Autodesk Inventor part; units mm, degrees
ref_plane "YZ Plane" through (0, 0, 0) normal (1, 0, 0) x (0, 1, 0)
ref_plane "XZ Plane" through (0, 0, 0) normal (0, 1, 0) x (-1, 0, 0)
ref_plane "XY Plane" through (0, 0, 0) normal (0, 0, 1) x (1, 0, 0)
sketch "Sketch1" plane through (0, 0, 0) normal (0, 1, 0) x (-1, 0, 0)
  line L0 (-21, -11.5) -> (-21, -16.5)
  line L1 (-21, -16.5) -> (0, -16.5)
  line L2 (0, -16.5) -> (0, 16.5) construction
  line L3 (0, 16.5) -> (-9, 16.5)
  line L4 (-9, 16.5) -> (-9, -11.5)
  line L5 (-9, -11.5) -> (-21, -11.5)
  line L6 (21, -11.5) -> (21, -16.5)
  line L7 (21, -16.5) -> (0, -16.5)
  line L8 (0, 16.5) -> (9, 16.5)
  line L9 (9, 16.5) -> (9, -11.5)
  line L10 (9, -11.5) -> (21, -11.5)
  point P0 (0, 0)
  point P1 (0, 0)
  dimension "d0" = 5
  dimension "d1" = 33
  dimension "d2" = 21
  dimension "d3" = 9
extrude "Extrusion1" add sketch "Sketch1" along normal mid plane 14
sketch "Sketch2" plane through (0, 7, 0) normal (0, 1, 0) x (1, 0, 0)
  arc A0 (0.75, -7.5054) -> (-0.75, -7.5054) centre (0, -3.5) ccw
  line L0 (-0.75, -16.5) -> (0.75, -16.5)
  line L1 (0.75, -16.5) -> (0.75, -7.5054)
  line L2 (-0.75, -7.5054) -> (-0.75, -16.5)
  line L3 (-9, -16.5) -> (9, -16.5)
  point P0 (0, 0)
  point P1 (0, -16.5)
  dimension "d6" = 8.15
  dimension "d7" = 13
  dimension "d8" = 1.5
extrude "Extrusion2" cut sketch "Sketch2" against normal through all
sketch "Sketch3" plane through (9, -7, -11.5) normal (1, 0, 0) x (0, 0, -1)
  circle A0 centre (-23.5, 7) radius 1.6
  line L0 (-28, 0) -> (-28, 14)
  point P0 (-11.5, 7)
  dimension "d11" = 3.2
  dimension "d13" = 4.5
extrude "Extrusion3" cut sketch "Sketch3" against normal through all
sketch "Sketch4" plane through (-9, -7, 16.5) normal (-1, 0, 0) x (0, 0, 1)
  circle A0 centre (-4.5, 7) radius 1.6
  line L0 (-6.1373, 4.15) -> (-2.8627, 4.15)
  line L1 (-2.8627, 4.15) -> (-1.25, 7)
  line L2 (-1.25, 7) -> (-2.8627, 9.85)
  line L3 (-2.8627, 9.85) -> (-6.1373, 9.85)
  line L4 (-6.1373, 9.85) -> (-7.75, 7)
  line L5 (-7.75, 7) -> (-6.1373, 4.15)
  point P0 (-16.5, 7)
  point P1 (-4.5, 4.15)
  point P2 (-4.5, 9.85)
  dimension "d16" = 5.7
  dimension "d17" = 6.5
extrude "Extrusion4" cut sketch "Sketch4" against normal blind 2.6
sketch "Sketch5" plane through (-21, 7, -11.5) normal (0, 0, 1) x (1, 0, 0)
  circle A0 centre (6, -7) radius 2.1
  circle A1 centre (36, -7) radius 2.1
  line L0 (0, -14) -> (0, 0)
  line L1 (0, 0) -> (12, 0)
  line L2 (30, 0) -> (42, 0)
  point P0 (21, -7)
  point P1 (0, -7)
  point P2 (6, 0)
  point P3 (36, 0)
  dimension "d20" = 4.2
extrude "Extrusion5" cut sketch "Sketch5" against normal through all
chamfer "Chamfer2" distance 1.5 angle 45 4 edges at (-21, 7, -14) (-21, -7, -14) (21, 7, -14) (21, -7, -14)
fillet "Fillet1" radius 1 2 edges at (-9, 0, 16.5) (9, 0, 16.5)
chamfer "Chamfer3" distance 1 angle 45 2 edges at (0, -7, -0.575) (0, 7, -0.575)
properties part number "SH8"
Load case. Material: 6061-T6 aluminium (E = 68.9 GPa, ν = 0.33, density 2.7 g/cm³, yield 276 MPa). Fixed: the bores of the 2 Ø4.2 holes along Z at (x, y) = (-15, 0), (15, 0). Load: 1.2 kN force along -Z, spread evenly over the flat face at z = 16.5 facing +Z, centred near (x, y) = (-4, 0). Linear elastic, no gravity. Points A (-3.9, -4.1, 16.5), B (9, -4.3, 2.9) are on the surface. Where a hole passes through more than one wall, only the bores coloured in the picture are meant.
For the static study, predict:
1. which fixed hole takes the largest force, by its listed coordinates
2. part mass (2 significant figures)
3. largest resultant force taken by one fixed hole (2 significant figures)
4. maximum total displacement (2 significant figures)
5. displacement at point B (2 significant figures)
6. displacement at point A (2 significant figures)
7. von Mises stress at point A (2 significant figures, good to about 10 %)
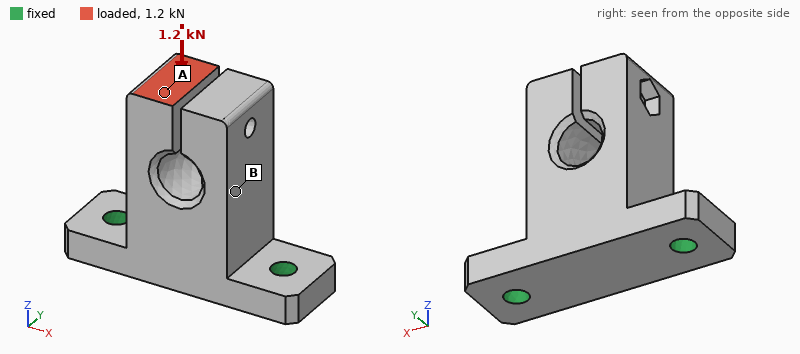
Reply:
(-15, 0)
23 g
860 N
28 µm
5.0 µm
24 µm
13 MPa
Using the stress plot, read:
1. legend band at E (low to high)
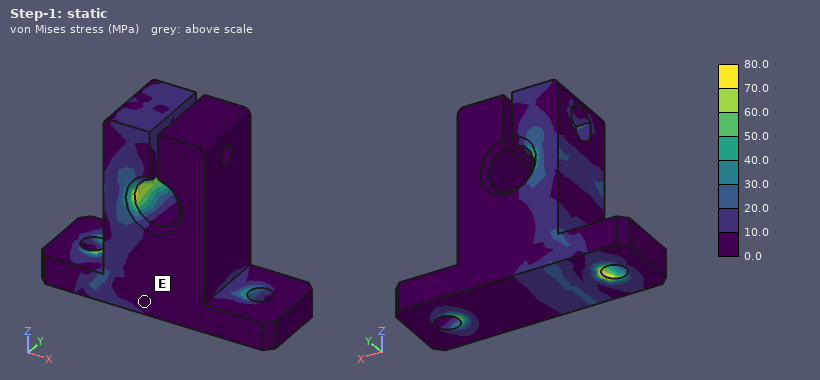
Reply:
0.0 to 10.0 MPa
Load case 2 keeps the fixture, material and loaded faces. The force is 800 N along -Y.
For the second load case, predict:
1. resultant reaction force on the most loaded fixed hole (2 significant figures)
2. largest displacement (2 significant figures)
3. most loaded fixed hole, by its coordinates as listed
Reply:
510 N
0.25 mm
(-15, 0)
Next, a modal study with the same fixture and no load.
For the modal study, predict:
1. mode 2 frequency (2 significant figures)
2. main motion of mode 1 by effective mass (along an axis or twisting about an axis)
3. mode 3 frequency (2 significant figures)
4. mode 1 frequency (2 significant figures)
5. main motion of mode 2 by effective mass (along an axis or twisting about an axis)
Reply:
7500 Hz
along Y
9600 Hz
4200 Hz
along X
